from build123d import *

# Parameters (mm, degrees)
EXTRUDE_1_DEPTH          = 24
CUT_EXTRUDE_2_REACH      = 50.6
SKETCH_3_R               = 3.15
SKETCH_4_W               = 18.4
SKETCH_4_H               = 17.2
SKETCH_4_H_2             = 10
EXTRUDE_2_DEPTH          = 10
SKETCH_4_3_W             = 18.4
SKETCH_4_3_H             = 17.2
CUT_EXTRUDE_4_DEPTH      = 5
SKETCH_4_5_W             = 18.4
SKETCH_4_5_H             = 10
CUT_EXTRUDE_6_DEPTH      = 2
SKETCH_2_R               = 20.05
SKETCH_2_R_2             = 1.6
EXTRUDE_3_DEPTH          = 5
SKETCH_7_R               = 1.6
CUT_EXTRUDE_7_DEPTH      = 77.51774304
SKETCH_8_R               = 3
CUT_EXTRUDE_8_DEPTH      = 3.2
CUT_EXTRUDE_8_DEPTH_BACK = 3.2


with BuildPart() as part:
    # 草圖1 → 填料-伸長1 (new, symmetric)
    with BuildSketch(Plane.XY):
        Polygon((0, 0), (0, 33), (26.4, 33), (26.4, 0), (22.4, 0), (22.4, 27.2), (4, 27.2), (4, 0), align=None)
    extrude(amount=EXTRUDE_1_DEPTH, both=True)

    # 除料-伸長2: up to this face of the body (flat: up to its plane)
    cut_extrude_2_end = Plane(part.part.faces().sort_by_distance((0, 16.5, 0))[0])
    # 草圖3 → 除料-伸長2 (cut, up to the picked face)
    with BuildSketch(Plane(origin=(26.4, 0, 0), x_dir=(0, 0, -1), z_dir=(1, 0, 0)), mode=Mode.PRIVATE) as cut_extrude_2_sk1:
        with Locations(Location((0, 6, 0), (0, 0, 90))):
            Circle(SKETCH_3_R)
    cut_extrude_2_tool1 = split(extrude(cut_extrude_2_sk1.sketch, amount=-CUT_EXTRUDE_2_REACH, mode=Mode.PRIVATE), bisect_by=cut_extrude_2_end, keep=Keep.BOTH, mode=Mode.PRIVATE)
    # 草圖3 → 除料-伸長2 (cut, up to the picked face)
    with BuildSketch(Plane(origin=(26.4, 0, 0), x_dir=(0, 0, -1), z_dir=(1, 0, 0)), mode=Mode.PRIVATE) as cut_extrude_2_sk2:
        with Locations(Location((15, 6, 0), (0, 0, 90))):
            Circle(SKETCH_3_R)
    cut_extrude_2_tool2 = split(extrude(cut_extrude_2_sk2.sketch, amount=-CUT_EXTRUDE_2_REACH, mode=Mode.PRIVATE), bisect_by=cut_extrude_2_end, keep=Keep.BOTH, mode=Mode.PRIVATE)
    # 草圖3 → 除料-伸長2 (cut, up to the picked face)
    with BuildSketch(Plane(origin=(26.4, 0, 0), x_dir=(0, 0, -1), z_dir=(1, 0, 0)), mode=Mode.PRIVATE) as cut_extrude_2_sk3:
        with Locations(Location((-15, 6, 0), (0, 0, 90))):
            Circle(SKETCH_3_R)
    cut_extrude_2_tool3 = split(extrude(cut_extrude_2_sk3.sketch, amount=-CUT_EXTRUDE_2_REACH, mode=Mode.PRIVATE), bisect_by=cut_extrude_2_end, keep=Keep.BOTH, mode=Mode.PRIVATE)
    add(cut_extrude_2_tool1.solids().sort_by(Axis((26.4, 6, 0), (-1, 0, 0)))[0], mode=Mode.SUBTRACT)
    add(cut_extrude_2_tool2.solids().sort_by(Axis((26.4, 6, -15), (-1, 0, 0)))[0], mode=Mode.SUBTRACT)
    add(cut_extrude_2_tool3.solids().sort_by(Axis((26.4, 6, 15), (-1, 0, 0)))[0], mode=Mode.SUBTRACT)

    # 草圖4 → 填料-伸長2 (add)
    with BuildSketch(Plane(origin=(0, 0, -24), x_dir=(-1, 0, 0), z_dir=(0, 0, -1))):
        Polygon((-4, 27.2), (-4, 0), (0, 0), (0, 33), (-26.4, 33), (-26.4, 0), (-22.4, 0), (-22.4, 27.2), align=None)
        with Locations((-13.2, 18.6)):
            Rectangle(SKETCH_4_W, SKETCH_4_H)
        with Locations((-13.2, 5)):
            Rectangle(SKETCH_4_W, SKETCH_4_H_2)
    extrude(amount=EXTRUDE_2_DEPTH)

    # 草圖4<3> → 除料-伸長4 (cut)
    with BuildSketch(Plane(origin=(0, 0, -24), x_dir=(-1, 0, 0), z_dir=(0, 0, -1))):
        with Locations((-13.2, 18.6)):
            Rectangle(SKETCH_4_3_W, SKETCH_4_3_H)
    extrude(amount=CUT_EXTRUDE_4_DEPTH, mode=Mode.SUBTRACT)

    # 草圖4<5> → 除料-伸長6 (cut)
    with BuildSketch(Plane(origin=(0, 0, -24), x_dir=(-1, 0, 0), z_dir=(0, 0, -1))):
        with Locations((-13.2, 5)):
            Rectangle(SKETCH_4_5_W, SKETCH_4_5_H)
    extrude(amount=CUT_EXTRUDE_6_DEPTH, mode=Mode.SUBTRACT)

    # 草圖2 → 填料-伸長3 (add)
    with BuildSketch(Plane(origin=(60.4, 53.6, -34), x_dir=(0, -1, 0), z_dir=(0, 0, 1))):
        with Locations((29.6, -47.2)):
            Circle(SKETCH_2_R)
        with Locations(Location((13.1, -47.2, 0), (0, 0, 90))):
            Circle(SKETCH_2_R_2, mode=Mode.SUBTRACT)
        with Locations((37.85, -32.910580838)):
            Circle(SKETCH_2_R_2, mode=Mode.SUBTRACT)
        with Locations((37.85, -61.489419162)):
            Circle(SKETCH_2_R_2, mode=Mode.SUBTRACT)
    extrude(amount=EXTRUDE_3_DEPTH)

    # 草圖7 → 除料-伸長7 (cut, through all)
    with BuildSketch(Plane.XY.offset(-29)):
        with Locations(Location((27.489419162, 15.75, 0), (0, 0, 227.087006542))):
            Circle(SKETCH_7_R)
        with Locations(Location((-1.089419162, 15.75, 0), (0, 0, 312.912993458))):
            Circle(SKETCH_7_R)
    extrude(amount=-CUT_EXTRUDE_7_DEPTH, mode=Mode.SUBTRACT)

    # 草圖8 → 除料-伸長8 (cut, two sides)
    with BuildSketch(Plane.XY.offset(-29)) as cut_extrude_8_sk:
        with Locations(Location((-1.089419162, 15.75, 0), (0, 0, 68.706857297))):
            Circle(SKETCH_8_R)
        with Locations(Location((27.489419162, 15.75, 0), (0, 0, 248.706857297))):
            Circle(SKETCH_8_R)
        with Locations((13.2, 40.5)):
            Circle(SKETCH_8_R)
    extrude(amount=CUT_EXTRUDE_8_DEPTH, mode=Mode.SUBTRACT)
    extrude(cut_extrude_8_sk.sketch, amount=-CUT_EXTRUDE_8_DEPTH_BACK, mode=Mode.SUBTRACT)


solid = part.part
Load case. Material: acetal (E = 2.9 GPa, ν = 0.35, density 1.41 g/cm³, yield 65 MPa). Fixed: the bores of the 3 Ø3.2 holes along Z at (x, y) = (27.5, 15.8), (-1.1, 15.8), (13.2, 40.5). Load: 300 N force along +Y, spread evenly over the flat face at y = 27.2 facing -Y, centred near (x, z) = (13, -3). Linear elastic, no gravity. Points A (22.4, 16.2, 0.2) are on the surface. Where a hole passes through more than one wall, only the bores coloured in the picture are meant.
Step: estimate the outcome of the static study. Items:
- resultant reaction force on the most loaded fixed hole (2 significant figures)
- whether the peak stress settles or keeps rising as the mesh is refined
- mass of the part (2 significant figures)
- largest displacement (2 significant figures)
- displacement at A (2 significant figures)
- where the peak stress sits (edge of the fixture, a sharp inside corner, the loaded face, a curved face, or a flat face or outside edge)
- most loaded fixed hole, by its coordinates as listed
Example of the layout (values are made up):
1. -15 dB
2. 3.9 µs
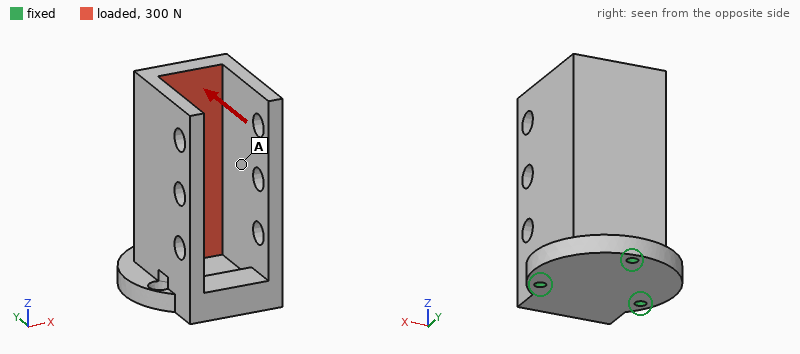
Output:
1. 470 N
2. keeps rising
3. 37 g
4. 0.68 mm
5. 0.37 mm
6. edge of the fixture
7. (13.2, 40.5)
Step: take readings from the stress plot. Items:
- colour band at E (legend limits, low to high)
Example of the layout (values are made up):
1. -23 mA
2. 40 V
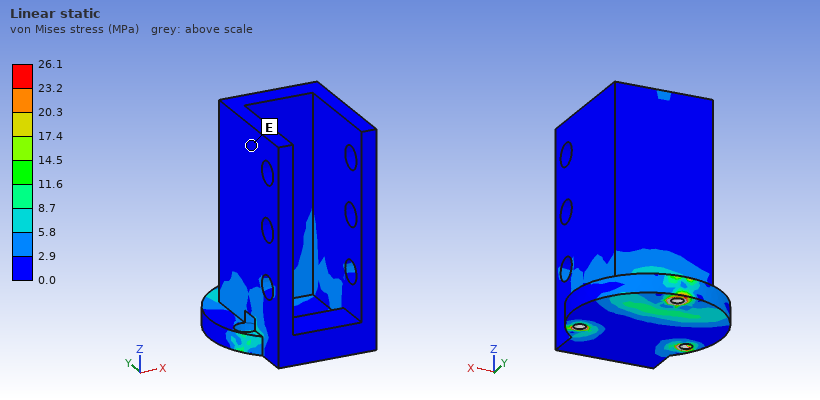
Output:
1. 0.0 to 2.9 MPa
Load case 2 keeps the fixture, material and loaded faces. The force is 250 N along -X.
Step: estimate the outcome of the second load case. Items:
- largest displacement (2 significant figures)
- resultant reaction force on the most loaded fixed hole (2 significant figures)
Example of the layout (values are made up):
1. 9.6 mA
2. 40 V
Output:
1. 0.86 mm
2. 310 N
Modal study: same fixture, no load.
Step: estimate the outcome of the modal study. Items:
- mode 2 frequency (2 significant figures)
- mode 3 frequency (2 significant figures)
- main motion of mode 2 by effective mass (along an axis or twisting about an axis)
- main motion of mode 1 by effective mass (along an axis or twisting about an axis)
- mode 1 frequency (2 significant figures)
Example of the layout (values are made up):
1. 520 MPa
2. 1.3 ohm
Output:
1. 770 Hz
2. 1300 Hz
3. along Y
4. along X
5. 630 Hz
